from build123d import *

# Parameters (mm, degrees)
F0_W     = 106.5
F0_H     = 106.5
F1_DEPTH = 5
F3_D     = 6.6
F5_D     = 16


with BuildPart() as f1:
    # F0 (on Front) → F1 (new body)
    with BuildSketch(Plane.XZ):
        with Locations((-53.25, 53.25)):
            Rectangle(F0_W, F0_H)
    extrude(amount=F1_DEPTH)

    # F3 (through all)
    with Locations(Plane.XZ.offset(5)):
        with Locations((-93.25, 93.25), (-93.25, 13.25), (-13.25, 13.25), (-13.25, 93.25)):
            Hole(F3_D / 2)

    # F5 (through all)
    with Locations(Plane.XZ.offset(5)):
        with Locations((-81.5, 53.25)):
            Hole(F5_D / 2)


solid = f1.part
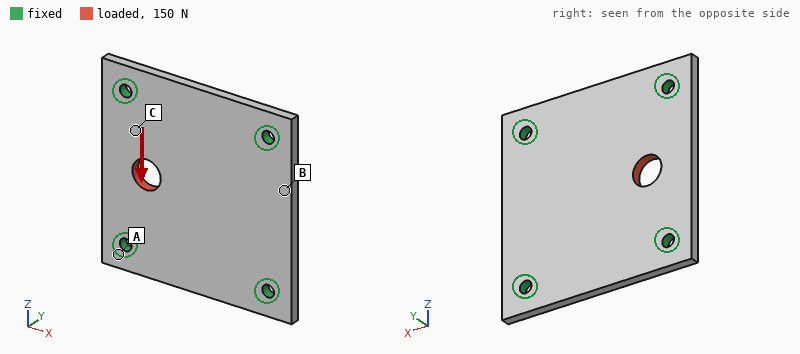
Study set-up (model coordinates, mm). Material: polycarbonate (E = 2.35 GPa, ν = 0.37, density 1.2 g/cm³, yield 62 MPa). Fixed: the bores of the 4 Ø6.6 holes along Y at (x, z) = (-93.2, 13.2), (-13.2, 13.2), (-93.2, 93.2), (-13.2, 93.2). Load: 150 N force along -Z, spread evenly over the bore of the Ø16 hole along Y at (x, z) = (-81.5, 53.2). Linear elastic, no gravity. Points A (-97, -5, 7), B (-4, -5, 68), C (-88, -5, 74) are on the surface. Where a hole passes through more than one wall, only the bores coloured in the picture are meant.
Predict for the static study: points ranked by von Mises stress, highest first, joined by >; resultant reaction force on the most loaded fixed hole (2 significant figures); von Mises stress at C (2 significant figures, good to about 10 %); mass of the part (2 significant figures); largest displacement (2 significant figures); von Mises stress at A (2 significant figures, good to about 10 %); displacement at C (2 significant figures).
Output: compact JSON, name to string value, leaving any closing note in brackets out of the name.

{"points ranked by von Mises stress, highest first, joined by >": "C > A > B", "resultant reaction force on the most loaded fixed hole": "60 N", "von Mises stress at C": "0.53 MPa", "mass of the part": "66 g", "largest displacement": "9.1 µm", "von Mises stress at A": "0.21 MPa", "displacement at C": "4.6 µm"}
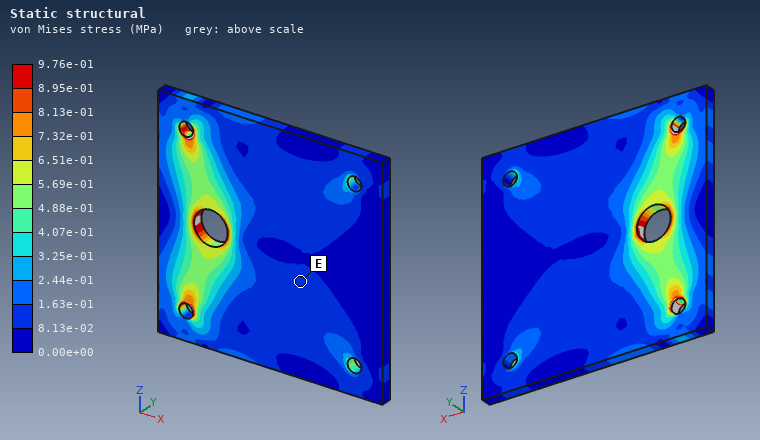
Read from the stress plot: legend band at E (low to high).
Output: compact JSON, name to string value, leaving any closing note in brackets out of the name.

{"legend band at E": "8.13e-02 to 1.63e-01 MPa"}
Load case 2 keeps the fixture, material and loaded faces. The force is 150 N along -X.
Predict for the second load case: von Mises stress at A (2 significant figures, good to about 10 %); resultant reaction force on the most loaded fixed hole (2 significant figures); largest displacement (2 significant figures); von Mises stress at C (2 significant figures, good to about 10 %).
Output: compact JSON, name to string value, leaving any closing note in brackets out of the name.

{"von Mises stress at A": "0.23 MPa", "resultant reaction force on the most loaded fixed hole": "44 N", "largest displacement": "16 µm", "von Mises stress at C": "0.35 MPa"}
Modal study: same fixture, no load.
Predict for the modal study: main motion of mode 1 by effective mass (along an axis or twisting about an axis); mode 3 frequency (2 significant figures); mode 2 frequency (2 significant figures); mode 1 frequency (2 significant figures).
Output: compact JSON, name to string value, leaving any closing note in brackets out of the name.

{"main motion of mode 1 by effective mass": "along Y", "mode 3 frequency": "1300 Hz", "mode 2 frequency": "1200 Hz", "mode 1 frequency": "810 Hz"}
